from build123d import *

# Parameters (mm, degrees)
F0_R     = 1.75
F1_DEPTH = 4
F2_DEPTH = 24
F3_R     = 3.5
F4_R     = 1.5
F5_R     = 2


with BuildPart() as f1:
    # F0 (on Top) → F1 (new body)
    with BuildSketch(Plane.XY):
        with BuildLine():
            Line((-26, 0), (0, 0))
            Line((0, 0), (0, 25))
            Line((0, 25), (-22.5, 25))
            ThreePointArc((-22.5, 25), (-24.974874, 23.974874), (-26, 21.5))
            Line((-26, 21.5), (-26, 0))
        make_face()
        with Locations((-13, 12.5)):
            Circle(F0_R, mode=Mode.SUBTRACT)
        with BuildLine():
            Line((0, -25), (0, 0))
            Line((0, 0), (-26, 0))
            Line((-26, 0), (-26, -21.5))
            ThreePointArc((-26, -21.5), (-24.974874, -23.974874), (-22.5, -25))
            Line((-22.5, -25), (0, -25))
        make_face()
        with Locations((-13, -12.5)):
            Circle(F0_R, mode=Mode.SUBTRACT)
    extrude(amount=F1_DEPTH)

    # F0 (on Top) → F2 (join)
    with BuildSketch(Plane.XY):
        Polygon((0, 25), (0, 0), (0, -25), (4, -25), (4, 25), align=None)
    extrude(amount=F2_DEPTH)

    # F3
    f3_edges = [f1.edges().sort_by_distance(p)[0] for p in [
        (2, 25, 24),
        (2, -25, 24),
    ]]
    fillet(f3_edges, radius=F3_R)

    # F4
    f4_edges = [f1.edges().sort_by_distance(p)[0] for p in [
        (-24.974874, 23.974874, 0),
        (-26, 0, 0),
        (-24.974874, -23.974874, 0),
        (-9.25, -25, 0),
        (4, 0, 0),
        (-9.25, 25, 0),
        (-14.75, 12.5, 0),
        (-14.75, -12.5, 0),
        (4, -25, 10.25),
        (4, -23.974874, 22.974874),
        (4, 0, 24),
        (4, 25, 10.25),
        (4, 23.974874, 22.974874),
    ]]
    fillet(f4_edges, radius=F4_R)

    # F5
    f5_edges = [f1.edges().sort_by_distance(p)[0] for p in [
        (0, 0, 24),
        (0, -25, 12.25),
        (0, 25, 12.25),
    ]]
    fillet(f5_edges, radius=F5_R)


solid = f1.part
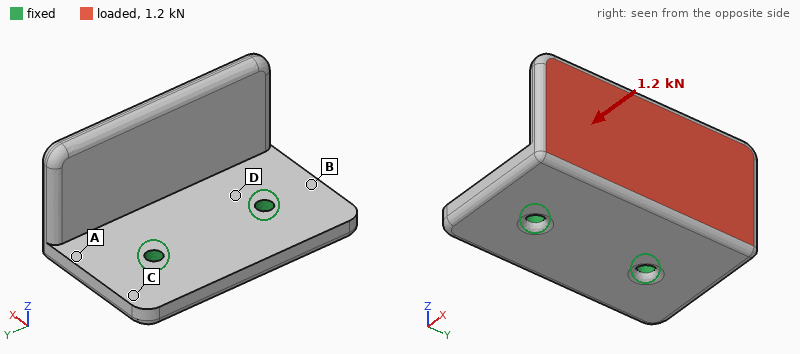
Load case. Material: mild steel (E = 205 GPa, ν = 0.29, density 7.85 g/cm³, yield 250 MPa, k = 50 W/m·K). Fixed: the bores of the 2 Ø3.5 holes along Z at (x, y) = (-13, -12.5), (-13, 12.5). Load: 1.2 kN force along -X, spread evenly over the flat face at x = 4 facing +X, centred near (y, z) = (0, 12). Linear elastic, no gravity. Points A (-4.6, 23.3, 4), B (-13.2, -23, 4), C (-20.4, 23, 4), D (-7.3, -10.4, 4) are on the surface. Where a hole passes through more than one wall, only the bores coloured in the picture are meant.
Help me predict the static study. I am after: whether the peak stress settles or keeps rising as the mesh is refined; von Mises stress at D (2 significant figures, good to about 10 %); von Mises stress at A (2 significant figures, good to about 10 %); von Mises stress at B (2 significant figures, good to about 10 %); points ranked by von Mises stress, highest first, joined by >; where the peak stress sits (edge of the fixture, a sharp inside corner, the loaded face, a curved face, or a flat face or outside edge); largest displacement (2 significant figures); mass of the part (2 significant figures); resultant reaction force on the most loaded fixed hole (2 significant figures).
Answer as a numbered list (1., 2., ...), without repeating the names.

1. keeps rising
2. 100 MPa
3. 82 MPa
4. 44 MPa
5. D > A > B > C
6. edge of the fixture
7. 0.11 mm
8. 76 g
9. 610 N
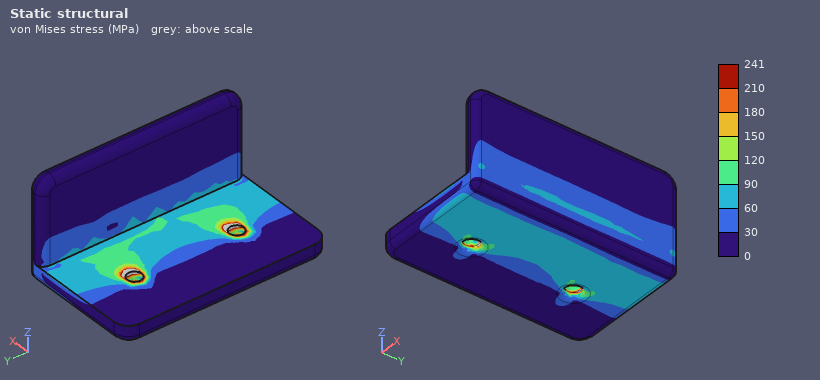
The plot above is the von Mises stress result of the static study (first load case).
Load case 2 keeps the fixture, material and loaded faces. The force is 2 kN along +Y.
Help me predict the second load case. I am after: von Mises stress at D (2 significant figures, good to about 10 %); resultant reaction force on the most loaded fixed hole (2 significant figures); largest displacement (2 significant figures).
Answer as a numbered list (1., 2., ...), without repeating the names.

1. 86 MPa
2. 1.7 kN
3. 48 µm
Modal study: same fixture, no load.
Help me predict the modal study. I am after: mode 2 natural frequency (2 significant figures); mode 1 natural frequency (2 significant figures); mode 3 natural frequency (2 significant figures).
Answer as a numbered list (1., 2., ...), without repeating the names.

1. 4700 Hz
2. 2800 Hz
3. 7700 Hz
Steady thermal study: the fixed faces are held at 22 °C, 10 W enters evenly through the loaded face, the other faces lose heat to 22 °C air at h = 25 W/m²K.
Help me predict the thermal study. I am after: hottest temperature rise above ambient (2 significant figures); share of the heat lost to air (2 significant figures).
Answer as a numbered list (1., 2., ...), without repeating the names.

1. 25 K
2. 13 %
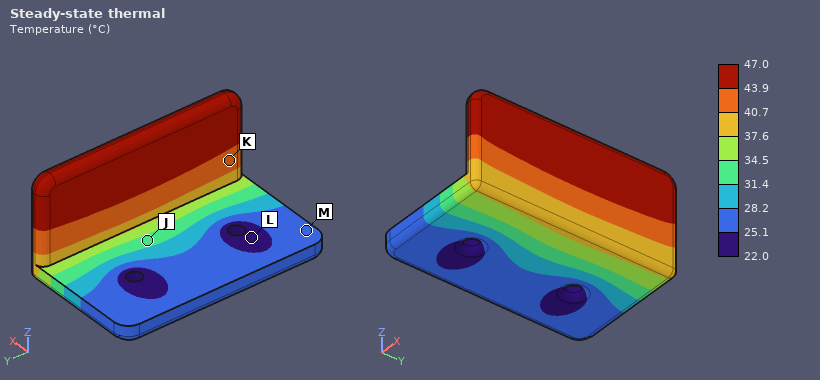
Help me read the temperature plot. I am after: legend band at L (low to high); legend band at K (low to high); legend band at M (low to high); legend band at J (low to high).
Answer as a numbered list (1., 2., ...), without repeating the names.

1. 22.0 to 25.1 °C
2. 40.7 to 43.9 °C
3. 25.1 to 28.2 °C
4. 31.4 to 34.5 °C
